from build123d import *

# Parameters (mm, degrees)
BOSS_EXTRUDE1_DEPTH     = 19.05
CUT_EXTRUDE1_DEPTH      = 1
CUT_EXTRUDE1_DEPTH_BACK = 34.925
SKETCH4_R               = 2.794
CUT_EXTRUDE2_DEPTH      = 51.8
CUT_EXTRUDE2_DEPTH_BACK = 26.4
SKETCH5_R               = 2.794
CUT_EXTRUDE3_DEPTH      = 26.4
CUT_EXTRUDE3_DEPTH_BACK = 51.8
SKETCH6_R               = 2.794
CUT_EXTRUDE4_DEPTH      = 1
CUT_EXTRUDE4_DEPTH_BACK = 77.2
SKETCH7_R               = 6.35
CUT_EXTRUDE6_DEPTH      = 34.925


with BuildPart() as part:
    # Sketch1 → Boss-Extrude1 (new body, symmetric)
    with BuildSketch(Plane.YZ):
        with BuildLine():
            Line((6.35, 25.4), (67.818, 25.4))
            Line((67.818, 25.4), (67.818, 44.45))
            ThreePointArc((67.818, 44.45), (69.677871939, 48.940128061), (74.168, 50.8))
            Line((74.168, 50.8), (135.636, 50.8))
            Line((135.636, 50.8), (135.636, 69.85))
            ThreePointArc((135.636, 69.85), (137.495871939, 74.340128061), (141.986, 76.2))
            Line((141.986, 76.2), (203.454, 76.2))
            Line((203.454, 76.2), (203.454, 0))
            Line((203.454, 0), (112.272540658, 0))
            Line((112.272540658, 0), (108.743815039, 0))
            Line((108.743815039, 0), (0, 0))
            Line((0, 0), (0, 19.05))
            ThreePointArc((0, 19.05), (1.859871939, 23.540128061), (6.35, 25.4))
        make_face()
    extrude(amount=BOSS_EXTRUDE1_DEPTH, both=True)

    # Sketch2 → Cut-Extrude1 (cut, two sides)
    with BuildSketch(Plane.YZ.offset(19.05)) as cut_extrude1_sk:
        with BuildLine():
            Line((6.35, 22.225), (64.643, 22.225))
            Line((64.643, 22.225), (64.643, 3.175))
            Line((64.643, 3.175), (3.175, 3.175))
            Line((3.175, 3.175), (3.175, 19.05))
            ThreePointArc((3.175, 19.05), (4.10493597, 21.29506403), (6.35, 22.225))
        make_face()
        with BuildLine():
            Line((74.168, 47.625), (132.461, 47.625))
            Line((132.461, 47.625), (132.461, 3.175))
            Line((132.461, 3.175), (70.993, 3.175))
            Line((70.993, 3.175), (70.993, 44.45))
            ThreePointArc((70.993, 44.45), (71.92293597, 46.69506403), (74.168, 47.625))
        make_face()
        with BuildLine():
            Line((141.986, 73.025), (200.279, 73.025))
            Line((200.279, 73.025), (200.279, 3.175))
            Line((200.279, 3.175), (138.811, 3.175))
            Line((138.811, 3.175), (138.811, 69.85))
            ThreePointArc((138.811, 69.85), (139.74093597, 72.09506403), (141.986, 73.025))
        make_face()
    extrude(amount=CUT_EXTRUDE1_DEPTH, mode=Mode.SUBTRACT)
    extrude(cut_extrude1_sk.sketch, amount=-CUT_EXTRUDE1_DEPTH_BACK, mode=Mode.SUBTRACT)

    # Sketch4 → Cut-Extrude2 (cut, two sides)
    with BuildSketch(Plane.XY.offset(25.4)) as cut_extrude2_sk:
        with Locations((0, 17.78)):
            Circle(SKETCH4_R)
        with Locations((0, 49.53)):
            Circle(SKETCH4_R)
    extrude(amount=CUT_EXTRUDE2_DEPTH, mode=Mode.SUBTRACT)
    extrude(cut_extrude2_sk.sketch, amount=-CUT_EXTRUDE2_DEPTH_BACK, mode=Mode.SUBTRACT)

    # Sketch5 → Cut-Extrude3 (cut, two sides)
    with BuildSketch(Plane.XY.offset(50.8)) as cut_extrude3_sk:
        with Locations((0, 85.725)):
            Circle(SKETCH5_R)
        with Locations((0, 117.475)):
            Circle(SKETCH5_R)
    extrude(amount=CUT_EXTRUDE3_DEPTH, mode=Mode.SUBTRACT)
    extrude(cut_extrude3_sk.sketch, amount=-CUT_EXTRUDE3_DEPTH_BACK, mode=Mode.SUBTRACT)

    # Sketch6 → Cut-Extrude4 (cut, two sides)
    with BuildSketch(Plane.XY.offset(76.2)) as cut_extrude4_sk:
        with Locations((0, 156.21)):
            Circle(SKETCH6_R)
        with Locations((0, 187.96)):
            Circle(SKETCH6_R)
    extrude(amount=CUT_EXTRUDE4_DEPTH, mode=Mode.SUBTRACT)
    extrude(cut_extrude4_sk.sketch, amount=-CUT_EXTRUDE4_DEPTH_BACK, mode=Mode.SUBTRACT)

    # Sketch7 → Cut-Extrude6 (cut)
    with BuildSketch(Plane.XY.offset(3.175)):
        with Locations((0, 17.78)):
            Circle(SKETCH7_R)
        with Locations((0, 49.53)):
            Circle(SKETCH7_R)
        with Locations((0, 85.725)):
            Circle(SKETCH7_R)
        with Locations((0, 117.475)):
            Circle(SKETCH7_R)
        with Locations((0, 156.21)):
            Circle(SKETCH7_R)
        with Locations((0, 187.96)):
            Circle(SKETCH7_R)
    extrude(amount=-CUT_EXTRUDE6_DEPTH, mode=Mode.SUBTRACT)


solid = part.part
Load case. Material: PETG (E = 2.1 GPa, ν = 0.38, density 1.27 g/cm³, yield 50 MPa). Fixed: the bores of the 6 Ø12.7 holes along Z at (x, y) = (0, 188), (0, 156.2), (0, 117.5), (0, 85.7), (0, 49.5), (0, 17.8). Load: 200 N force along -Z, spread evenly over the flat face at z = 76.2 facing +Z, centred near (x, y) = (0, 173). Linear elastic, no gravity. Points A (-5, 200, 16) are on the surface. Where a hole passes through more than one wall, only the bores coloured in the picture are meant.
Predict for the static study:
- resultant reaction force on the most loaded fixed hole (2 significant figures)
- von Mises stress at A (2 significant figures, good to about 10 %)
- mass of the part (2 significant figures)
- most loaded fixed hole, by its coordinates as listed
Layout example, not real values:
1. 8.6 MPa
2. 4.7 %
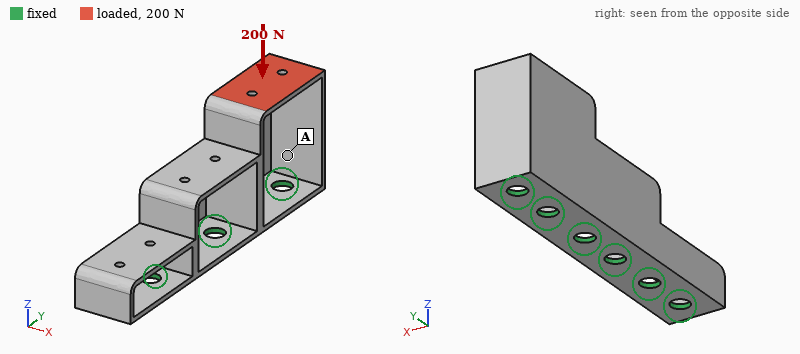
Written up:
1. 100 N
2. 1.5 MPa
3. 130 g
4. (0, 188)
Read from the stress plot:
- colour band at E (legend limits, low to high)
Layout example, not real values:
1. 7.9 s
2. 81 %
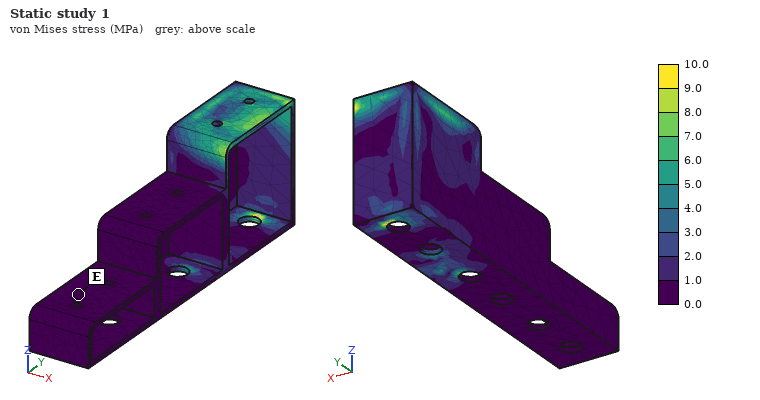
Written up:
1. 0.0 to 1.0 MPa
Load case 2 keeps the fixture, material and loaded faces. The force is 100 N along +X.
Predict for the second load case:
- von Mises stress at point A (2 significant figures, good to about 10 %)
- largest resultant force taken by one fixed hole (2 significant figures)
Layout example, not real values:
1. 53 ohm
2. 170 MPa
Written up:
1. 2.3 MPa
2. 59 N
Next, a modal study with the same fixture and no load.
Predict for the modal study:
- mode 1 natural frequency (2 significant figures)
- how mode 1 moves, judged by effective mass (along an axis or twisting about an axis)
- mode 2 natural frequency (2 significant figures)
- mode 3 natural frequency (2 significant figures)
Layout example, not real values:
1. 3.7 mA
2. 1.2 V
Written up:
1. 240 Hz
2. along X
3. 400 Hz
4. 680 Hz
